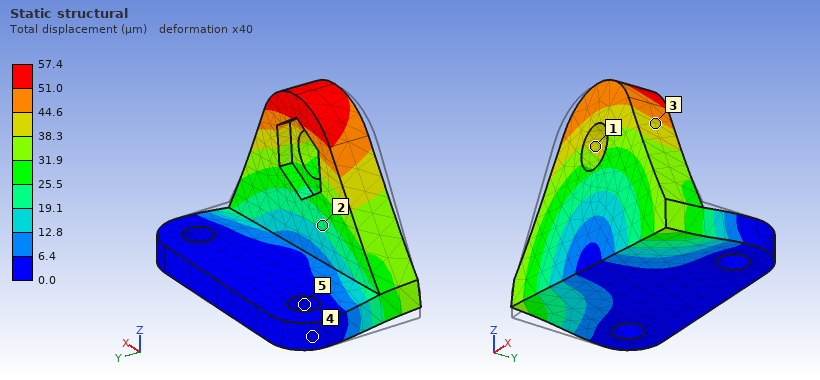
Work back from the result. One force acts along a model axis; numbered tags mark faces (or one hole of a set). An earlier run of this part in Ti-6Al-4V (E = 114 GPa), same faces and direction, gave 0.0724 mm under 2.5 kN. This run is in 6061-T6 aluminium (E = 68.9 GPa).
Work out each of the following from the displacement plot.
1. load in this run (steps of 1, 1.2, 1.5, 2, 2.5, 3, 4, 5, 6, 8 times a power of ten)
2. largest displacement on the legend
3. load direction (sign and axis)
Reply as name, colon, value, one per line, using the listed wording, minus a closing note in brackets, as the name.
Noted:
load in this run: 1.2 kN
largest displacement on the legend: 57.4 µm
load direction: +X
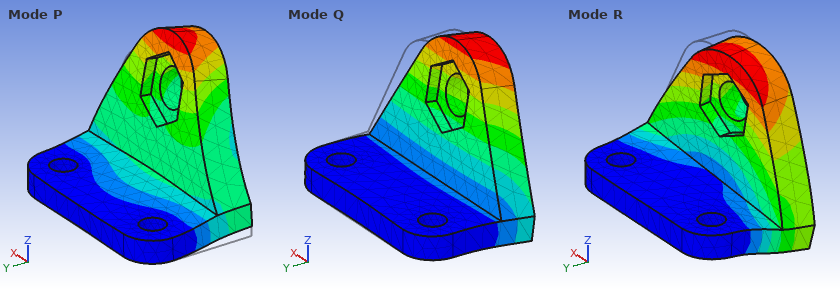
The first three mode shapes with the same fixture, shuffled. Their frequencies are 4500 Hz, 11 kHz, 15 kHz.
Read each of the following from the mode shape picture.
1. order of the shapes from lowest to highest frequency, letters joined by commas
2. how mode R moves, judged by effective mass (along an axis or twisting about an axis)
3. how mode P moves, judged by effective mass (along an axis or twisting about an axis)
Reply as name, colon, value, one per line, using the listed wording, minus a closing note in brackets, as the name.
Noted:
order of the shapes from lowest to highest frequency, letters joined by commas: Q, R, P
how mode R moves, judged by effective mass: along X
how mode P moves, judged by effective mass: along Z
